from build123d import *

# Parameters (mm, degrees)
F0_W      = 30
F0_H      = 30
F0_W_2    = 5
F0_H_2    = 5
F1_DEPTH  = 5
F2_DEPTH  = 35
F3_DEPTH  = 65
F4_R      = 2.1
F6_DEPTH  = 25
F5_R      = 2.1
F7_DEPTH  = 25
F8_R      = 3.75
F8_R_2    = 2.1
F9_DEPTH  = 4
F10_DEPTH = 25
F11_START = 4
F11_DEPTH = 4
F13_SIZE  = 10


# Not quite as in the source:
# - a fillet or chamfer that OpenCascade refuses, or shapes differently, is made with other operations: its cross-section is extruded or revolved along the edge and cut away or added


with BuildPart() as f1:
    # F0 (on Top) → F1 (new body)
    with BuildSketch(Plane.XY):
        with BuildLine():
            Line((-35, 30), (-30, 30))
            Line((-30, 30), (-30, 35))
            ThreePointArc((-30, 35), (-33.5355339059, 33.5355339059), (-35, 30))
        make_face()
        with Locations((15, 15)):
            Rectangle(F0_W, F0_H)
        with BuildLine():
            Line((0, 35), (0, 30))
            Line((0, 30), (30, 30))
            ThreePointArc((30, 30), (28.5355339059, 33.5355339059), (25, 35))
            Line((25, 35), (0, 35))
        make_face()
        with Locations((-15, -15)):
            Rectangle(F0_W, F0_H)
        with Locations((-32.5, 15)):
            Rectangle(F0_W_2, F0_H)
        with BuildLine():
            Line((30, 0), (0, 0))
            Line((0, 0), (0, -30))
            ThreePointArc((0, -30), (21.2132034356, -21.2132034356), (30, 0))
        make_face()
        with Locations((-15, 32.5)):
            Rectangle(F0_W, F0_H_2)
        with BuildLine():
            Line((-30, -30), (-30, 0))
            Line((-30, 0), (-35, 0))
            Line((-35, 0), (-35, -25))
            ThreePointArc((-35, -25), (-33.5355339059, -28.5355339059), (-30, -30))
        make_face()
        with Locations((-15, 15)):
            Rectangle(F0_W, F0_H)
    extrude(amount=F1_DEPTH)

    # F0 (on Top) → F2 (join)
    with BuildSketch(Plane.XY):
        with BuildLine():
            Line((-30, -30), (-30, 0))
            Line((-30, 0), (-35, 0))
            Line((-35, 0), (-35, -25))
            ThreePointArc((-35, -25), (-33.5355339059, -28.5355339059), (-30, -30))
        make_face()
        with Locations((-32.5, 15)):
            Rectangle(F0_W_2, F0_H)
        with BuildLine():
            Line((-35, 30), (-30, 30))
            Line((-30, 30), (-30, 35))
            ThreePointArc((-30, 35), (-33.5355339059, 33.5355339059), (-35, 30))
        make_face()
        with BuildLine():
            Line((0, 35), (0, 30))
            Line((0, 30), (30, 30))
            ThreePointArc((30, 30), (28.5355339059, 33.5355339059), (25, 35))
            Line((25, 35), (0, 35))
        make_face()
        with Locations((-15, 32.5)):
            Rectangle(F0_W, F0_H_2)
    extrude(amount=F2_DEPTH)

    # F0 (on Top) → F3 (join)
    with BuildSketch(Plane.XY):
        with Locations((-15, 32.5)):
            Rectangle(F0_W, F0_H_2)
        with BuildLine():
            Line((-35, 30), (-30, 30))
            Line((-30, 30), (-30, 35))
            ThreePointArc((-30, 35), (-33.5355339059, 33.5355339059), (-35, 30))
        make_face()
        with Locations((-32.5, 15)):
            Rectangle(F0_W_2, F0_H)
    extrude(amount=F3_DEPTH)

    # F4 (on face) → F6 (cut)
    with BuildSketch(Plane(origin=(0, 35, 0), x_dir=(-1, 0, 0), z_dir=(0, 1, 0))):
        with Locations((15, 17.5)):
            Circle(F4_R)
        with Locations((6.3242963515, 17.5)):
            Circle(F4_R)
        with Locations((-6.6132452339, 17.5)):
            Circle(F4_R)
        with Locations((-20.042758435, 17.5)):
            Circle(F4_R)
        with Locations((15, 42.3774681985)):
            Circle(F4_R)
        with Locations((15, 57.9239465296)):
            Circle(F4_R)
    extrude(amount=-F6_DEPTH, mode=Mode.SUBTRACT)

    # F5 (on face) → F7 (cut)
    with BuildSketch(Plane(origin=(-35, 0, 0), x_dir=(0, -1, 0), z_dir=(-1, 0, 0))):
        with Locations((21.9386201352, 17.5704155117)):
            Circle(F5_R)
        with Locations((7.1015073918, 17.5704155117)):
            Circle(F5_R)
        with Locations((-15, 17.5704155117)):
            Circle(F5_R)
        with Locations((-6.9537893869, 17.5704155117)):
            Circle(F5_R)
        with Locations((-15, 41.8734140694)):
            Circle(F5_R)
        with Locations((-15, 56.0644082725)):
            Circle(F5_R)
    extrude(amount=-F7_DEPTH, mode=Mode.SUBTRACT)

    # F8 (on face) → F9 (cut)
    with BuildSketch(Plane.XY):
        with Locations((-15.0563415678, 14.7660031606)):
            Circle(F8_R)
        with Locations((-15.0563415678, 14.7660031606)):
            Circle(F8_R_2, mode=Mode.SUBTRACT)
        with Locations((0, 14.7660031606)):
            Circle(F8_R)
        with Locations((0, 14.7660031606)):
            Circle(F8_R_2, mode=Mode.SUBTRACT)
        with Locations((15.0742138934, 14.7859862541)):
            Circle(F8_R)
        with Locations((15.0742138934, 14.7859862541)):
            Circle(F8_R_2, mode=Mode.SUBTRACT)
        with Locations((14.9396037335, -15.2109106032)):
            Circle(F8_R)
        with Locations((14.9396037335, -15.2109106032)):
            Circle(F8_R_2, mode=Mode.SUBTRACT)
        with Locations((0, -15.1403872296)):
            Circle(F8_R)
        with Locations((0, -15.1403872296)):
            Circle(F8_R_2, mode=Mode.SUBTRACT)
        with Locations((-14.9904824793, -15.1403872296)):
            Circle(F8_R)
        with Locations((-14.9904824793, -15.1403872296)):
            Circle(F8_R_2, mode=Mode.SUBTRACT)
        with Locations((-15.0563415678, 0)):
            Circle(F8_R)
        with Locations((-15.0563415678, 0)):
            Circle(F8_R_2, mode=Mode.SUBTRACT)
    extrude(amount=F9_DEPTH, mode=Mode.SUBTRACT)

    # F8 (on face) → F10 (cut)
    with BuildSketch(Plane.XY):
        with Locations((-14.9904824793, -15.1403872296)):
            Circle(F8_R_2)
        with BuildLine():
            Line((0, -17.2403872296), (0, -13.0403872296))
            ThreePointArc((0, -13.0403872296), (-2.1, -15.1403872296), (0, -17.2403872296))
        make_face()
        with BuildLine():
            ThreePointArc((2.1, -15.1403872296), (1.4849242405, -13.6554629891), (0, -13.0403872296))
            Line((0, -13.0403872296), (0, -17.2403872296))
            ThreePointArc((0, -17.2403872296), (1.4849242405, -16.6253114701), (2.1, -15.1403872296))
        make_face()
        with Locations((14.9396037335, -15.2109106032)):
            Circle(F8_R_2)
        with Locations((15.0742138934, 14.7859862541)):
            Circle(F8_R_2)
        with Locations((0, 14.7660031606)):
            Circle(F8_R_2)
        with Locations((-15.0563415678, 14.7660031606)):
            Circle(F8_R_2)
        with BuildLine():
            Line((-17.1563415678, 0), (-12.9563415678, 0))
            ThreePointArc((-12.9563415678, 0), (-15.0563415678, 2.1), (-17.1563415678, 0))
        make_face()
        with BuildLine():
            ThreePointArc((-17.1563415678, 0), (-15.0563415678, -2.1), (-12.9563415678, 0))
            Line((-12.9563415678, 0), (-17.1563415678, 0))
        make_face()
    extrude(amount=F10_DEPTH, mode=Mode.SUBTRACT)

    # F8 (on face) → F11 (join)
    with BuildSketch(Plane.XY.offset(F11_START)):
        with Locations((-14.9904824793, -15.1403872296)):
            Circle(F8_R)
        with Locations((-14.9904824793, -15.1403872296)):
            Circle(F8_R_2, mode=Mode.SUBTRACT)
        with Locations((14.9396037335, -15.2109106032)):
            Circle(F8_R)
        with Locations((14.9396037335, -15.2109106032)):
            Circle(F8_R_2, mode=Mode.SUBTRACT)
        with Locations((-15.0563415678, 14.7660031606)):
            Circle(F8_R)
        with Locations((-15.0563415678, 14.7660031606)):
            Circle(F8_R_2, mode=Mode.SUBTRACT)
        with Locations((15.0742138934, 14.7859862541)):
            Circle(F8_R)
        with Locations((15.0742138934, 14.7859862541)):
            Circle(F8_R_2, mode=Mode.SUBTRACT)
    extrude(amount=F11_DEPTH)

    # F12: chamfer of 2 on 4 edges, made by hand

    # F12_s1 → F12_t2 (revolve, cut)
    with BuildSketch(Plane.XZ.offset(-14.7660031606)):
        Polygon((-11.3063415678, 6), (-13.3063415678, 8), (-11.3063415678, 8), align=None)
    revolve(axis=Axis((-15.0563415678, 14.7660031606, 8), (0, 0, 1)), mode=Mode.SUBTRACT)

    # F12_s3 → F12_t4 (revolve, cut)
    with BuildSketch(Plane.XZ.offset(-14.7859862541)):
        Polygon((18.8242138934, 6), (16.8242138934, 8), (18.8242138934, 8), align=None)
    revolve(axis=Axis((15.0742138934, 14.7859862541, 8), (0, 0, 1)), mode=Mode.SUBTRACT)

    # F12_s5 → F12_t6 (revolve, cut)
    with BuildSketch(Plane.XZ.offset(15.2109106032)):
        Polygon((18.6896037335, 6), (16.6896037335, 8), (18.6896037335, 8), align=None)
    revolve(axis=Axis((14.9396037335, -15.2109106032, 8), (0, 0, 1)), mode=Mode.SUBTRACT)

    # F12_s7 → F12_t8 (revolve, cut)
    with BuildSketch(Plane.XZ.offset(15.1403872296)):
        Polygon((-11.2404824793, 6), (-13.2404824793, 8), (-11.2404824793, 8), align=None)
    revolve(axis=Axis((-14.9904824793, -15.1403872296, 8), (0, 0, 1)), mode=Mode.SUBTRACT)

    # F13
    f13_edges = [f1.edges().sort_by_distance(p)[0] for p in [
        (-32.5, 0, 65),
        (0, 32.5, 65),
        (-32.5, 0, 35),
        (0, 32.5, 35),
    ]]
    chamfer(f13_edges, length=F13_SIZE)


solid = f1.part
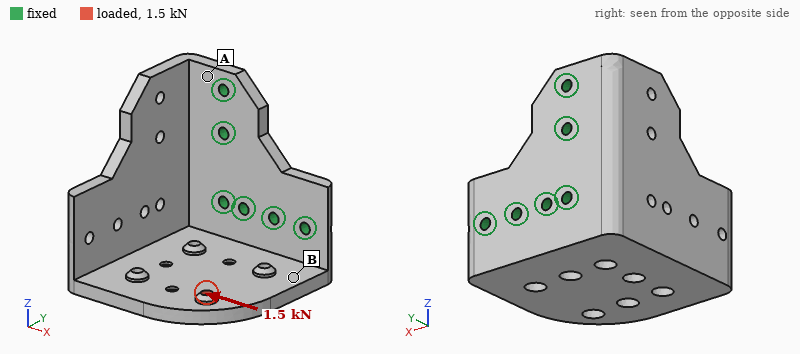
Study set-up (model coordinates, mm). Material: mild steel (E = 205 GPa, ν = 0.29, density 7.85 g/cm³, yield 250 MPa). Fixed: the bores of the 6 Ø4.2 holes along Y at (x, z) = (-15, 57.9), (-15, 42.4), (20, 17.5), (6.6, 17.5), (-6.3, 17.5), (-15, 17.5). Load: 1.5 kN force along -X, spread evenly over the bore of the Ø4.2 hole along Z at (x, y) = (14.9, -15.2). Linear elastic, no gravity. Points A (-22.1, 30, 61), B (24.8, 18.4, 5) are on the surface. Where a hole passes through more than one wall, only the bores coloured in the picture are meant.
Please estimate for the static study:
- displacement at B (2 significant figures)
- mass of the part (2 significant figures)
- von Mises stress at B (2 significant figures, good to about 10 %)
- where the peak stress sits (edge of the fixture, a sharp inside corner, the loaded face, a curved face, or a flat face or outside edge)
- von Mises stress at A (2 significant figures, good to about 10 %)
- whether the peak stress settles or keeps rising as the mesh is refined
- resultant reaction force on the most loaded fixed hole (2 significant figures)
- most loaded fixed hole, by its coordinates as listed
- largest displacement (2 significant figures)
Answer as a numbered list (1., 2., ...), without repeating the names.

1. 40 µm
2. 360 g
3. 53 MPa
4. edge of the fixture
5. 21 MPa
6. keeps rising
7. 2.1 kN
8. (-15, 17.5)
9. 88 µm
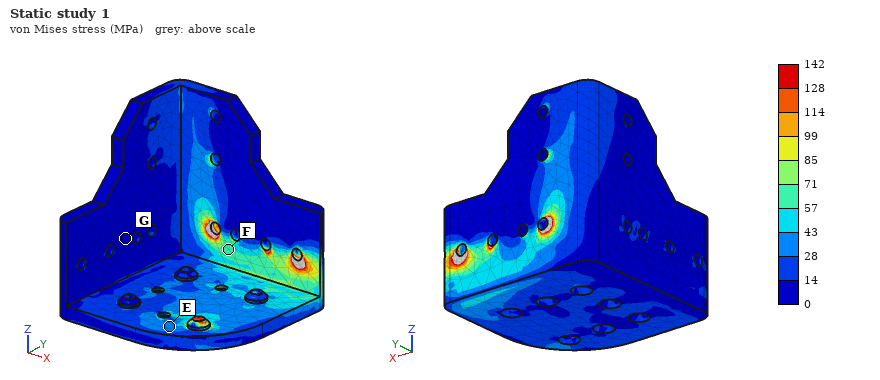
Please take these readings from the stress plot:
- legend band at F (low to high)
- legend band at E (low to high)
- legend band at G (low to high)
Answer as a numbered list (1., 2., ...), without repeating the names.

1. 57 to 71 MPa
2. 28 to 43 MPa
3. 0 to 14 MPa
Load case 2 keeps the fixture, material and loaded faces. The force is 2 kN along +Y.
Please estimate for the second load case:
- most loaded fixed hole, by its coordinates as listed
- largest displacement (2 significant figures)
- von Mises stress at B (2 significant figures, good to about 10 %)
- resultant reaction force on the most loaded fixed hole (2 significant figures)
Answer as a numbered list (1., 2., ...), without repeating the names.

1. (20, 17.5)
2. 46 µm
3. 53 MPa
4. 1.1 kN
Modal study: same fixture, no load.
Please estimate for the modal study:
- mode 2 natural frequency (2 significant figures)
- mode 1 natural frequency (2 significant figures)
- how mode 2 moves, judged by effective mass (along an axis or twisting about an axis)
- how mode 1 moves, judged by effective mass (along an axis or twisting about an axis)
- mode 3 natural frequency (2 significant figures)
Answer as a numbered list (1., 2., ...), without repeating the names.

1. 1900 Hz
2. 1600 Hz
3. along X
4. along Z
5. 3300 Hz
